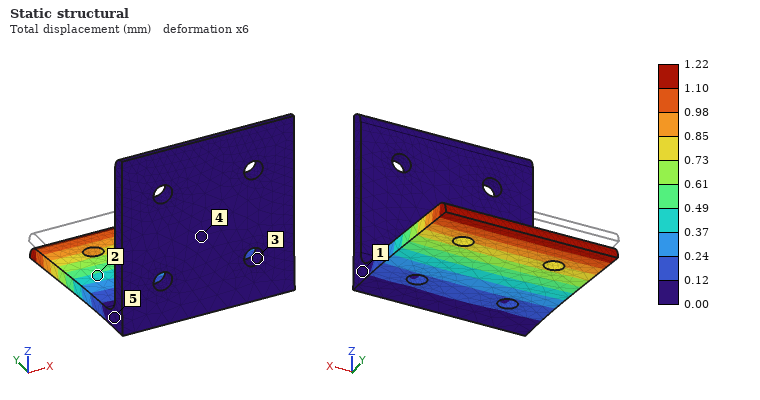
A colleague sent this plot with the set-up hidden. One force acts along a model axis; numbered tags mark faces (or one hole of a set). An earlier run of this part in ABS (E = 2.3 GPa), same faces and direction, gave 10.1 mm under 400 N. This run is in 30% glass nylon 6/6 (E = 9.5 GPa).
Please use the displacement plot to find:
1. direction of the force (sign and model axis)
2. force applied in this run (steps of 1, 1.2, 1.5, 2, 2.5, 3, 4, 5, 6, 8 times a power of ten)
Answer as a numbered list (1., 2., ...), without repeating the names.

1. -Z
2. 200 N
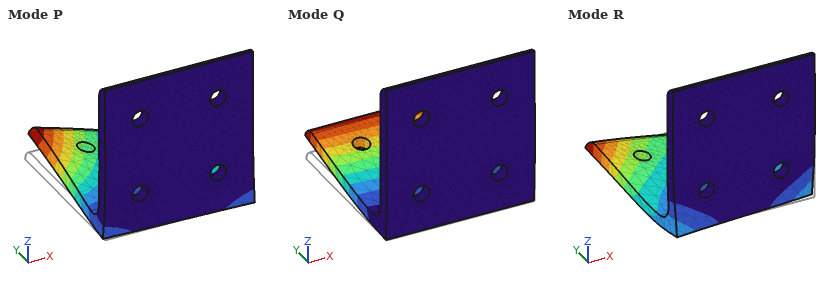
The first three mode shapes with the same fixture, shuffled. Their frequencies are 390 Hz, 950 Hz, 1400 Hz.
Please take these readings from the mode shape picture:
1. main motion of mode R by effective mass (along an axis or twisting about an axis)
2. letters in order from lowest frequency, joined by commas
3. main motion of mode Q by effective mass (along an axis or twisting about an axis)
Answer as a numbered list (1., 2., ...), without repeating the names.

1. along X
2. Q, P, R
3. along Z
